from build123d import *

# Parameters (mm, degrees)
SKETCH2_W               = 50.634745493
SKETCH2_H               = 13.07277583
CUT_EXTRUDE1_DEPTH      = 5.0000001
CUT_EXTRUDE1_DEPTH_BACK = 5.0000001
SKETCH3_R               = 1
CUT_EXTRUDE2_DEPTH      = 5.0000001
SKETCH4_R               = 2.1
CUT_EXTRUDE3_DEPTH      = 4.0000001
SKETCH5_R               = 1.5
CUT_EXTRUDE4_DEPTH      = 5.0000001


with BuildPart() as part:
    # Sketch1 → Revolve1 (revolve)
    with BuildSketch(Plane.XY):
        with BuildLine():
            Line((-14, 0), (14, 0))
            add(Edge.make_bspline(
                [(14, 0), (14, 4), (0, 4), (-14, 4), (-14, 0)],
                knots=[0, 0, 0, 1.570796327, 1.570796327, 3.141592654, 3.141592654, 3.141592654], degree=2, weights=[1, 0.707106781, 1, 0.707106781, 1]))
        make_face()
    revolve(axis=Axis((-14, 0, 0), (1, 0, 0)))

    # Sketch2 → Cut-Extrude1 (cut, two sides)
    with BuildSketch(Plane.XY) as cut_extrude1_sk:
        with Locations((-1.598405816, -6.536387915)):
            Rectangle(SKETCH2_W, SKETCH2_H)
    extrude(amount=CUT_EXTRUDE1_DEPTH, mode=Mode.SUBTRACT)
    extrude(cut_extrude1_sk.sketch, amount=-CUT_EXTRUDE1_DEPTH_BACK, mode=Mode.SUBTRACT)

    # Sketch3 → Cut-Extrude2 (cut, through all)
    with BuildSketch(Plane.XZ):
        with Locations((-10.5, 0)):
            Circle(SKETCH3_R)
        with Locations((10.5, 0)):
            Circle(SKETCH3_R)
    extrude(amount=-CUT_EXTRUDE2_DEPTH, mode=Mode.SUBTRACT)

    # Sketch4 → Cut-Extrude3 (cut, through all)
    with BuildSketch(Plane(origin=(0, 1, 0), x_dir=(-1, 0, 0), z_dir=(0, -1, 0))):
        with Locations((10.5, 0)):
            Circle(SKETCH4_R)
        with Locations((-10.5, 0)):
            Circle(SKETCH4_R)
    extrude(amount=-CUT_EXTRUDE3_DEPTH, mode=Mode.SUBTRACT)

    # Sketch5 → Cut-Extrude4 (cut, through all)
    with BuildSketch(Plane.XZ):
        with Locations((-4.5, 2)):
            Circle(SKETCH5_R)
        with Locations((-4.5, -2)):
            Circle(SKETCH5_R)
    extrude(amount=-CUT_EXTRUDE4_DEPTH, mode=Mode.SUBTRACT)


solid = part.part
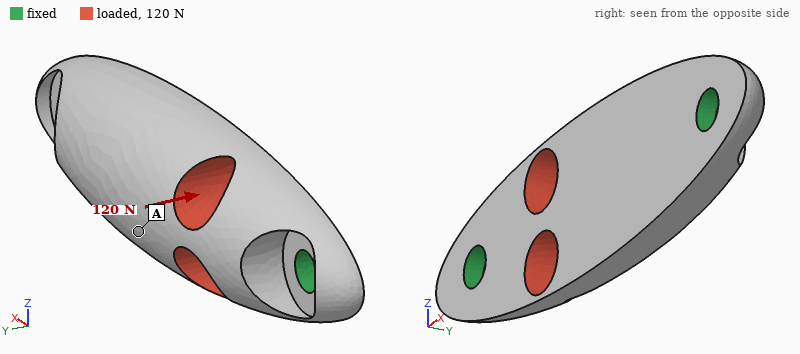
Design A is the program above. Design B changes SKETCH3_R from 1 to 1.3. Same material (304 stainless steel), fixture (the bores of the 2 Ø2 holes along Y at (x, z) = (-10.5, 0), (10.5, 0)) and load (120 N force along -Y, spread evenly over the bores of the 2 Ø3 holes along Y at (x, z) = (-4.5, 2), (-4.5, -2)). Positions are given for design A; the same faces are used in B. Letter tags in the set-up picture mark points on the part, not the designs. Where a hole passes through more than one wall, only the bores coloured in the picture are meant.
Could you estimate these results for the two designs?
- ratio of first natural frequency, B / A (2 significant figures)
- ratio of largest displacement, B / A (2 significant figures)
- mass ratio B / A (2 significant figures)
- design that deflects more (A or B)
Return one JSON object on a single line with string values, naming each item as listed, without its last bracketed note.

{"ratio of first natural frequency, B / A": "1.1", "ratio of largest displacement, B / A": "0.86", "mass ratio B / A": "0.99", "design that deflects more": "A"}
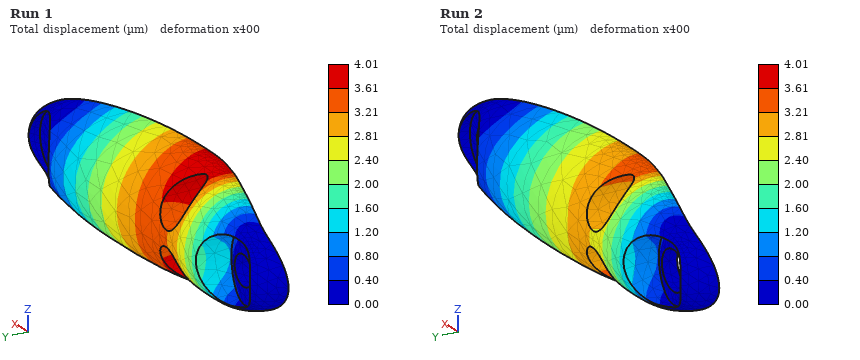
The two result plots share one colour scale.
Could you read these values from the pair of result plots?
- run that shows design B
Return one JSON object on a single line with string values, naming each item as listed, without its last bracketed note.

{"run that shows design B": "Run 2"}
